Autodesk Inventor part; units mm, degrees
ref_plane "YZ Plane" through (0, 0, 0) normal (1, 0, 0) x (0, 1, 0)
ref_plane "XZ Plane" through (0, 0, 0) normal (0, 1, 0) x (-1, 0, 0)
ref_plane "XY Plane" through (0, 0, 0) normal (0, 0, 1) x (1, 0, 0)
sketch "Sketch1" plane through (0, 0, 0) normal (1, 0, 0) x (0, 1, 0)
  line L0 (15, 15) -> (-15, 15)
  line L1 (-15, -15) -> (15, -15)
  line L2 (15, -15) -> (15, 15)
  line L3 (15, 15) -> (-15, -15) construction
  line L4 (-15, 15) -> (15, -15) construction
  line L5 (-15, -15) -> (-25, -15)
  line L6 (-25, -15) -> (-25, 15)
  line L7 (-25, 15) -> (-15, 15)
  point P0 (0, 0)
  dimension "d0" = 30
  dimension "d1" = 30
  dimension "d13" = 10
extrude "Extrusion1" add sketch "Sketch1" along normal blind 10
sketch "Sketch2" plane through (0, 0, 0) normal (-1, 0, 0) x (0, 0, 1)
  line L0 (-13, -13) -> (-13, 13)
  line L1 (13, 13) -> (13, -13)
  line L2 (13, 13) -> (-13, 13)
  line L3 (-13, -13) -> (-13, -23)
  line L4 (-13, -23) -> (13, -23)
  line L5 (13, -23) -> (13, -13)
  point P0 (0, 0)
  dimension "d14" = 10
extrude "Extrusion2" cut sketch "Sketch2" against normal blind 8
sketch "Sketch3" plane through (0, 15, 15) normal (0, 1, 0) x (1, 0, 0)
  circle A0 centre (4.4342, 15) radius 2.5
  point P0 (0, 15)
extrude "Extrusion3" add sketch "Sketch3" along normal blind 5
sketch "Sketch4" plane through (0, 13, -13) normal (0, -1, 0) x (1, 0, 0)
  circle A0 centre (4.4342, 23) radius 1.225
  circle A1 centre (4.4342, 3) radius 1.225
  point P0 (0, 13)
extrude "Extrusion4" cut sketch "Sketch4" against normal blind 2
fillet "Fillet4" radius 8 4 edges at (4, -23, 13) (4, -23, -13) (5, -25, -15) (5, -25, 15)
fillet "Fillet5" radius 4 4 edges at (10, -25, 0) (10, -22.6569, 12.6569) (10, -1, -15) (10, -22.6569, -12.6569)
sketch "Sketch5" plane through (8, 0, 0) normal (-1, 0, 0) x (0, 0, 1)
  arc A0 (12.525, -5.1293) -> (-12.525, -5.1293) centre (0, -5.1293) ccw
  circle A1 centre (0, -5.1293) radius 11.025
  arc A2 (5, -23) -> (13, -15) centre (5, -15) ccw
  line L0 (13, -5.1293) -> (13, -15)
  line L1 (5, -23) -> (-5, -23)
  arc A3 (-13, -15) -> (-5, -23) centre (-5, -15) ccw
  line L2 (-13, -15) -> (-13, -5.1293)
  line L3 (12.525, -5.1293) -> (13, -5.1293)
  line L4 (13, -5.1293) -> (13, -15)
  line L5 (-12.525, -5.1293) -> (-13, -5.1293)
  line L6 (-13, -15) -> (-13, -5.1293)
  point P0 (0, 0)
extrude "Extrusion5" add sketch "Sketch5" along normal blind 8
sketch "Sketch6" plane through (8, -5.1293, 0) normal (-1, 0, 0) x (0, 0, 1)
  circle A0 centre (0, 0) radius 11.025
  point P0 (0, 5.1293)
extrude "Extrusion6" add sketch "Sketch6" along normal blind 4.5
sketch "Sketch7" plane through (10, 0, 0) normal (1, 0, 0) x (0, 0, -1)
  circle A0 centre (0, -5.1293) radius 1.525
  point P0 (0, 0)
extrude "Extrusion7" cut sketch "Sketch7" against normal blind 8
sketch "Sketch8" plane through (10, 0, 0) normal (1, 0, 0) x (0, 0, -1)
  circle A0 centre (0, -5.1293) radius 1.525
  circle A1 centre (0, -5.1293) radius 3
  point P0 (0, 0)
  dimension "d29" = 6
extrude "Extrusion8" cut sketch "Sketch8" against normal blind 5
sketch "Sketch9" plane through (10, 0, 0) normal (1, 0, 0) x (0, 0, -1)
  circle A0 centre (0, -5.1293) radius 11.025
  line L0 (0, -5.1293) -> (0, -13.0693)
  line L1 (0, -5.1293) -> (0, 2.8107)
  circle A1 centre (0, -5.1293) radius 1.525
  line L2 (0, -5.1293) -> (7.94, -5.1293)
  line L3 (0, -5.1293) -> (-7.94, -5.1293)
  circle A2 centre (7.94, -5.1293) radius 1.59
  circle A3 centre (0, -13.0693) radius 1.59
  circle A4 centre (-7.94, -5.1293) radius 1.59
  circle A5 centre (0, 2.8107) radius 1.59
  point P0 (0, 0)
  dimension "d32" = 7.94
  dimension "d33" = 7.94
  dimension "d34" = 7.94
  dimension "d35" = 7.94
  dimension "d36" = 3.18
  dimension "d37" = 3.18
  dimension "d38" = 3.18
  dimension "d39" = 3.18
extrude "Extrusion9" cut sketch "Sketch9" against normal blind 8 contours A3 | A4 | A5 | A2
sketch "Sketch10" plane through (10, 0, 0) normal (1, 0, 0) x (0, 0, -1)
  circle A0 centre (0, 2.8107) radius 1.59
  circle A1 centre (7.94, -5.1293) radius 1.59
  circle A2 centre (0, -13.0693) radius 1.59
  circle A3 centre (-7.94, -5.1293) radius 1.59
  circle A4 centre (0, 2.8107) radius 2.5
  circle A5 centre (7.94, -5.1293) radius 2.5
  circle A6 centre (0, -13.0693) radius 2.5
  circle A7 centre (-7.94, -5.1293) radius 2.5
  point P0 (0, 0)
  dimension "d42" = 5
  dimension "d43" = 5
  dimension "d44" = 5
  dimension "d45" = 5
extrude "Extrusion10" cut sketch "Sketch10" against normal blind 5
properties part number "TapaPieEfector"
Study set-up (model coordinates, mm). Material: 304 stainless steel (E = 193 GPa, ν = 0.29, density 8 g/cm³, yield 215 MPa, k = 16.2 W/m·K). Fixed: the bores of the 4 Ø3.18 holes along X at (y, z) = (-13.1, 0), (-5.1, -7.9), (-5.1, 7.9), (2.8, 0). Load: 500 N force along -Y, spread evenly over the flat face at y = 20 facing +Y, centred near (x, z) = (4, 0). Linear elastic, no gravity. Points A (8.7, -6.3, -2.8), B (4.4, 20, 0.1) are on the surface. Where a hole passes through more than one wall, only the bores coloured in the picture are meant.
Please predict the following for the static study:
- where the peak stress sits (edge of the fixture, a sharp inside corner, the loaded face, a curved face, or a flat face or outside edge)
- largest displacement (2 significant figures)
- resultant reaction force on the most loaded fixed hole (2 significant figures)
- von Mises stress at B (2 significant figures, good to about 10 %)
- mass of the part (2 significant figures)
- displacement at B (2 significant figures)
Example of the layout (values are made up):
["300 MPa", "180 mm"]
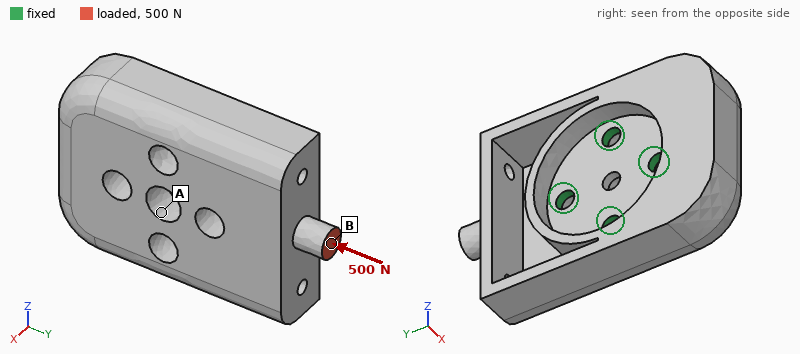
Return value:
["a curved face", "34 µm", "160 N", "26 MPa", "62 g", "29 µm"]
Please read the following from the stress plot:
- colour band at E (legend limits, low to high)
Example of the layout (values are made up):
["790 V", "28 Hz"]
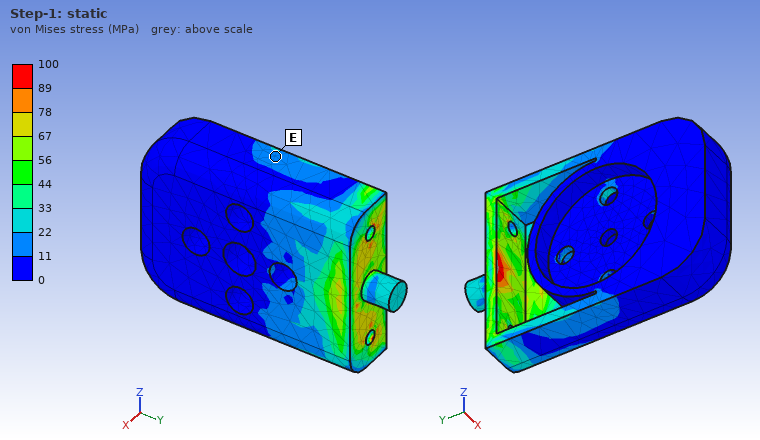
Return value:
["11 to 22 MPa"]
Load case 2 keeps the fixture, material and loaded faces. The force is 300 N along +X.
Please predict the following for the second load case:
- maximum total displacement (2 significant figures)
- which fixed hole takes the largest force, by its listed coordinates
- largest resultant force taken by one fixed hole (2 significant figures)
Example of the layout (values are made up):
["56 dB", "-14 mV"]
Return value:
["54 µm", "(2.8, 0)", "500 N"]
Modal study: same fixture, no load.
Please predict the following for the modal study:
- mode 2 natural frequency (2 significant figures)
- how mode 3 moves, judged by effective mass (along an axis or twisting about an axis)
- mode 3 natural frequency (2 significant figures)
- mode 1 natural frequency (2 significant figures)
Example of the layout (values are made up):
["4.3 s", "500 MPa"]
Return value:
["11 kHz", "along X", "14 kHz", "9100 Hz"]
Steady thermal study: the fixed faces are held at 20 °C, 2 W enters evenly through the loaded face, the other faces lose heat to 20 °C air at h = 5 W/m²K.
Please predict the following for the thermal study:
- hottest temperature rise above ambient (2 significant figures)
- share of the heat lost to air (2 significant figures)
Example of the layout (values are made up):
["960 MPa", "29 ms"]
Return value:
["73 K", "10 %"]
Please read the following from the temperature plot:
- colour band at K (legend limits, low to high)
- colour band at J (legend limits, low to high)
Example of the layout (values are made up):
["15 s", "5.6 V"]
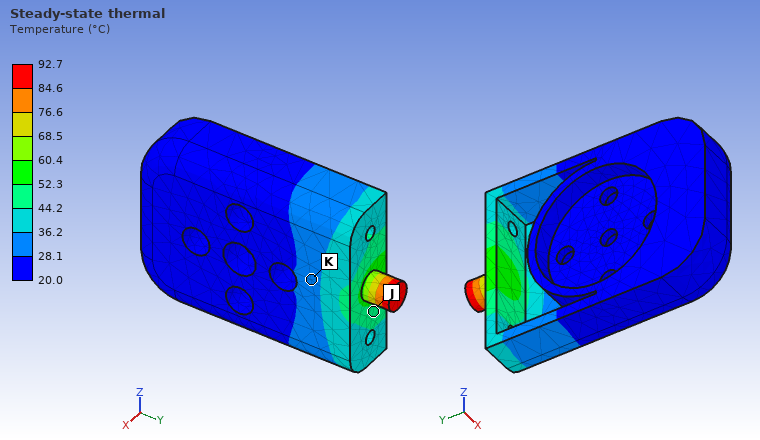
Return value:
["28.1 to 36.2 °C", "44.2 to 52.3 °C"]
